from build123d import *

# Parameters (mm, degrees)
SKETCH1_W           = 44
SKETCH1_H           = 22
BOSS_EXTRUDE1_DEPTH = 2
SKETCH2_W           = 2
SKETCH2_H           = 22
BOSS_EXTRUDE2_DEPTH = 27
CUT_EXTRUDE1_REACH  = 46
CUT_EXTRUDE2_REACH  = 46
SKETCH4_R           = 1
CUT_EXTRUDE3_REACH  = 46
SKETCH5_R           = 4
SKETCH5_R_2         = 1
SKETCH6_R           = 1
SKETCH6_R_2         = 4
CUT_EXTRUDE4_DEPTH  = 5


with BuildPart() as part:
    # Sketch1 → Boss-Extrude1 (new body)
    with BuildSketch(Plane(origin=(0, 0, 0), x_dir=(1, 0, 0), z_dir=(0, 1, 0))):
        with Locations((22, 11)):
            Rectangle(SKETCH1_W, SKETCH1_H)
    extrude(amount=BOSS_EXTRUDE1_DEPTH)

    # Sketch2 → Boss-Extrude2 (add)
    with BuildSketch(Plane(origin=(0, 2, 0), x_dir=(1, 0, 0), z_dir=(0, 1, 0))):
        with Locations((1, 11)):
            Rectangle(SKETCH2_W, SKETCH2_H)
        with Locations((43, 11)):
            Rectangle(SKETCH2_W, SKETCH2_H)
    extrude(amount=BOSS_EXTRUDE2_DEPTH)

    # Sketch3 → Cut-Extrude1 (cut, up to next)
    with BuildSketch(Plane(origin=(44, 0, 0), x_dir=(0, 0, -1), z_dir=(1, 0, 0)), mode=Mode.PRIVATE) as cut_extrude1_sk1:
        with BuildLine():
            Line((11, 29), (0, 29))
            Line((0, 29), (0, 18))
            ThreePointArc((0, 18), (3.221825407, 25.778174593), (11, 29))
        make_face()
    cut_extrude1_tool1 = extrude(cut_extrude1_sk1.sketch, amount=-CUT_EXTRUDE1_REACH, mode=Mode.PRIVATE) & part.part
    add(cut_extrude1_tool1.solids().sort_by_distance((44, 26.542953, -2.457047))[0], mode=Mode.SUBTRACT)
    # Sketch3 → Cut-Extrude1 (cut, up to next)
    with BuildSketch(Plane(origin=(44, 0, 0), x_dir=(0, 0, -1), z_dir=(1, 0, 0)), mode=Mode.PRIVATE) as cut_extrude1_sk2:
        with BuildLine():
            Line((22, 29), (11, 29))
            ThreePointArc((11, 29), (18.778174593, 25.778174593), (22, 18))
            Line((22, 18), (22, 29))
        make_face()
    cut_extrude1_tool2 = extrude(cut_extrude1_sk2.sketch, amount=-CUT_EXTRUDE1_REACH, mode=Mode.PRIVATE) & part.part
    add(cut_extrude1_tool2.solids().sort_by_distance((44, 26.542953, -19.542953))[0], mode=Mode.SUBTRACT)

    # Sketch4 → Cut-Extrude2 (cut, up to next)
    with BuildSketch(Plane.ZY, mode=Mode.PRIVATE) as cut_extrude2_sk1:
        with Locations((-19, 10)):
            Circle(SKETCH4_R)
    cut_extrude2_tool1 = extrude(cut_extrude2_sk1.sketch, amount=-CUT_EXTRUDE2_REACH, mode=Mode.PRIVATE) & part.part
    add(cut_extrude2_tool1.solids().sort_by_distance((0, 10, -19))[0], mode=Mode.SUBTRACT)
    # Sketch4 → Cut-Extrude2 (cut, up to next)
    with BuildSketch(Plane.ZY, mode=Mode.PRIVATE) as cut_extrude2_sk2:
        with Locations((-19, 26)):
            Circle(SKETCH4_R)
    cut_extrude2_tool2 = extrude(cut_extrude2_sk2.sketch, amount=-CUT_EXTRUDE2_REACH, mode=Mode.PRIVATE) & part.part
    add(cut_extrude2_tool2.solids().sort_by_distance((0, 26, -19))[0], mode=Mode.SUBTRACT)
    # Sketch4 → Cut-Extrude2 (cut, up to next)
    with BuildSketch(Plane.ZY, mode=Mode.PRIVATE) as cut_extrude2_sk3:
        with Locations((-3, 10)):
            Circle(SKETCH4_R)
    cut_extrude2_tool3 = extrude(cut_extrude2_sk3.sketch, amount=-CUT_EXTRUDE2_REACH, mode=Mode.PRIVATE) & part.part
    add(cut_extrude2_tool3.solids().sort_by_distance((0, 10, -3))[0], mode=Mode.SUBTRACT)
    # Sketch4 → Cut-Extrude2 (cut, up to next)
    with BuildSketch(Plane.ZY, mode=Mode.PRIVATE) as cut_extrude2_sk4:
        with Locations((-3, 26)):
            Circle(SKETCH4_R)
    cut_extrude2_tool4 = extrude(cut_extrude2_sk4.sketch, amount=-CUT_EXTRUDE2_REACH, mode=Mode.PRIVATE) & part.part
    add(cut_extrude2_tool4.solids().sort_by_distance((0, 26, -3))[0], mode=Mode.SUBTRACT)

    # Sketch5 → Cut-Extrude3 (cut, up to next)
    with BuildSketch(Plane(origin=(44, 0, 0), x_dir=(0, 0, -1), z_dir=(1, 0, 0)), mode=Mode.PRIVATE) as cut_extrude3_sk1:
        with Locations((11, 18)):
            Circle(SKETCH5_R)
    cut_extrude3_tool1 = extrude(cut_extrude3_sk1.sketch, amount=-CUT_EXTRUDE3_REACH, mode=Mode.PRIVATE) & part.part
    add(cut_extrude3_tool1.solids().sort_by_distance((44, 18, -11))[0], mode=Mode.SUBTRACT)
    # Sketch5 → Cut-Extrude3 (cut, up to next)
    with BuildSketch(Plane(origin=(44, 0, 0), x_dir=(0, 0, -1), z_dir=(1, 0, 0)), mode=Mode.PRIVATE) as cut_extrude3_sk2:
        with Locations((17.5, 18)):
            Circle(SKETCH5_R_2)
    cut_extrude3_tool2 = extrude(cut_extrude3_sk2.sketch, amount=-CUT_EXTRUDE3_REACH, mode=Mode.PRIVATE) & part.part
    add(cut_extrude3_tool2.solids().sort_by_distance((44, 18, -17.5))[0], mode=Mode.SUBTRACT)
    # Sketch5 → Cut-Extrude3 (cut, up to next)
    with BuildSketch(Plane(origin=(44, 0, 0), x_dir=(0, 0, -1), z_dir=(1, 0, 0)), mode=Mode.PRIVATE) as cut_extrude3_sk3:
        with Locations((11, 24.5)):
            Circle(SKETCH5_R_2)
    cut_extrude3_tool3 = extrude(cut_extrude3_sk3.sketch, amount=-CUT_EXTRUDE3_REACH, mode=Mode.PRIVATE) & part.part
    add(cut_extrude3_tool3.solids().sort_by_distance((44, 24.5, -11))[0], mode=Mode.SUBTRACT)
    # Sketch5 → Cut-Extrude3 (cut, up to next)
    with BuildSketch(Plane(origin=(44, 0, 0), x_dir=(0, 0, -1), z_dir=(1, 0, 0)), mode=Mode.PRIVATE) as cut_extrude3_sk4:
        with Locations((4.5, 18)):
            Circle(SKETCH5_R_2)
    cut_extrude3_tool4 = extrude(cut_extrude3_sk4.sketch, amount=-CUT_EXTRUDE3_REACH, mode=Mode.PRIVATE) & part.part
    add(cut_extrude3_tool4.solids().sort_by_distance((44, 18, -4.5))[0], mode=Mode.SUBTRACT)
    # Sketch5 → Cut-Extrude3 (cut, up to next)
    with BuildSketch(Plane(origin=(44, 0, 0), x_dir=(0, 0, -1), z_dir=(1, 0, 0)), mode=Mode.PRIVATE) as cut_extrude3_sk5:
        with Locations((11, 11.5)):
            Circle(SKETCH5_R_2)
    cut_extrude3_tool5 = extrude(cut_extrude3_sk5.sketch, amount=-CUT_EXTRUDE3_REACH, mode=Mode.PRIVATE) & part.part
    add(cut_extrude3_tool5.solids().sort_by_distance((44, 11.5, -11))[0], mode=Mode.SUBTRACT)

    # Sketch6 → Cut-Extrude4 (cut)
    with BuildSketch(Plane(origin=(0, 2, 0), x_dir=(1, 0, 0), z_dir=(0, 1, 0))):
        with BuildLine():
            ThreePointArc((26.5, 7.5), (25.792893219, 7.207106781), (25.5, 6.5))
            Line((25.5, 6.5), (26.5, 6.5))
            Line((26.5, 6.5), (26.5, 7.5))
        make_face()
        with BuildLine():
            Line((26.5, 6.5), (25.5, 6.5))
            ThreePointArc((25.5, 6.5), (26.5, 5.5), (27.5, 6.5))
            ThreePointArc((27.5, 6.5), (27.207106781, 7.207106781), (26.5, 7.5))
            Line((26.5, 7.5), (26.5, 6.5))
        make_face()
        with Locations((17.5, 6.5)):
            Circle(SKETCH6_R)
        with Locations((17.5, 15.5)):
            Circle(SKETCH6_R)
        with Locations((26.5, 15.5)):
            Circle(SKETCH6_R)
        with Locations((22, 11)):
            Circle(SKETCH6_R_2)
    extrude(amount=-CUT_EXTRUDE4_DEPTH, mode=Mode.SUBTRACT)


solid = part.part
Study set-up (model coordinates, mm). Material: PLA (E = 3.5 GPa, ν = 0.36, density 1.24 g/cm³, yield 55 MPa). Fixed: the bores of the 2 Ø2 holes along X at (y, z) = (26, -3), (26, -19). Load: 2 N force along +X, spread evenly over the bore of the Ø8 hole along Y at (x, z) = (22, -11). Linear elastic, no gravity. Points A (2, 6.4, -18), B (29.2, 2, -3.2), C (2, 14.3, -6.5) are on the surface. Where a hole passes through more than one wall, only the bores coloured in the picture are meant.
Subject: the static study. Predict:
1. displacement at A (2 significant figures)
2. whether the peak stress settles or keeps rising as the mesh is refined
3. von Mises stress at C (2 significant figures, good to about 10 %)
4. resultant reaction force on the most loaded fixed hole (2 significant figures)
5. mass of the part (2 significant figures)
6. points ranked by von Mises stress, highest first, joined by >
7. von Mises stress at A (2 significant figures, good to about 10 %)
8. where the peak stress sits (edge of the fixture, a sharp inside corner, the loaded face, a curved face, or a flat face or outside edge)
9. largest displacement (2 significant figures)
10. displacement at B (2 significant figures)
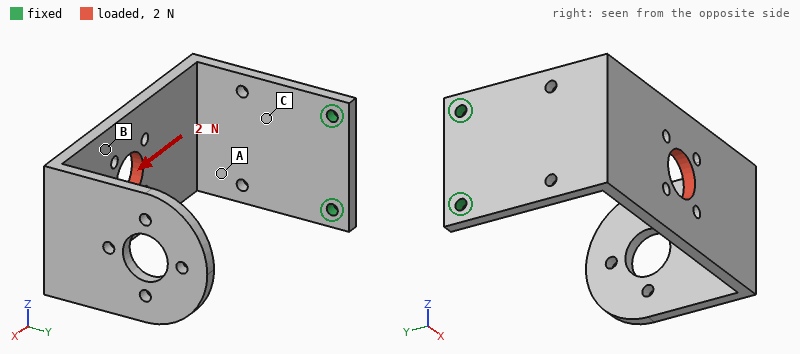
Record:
0.15 mm
keeps rising
1.7 MPa
1.0 N
4.9 g
C > A > B
0.77 MPa
edge of the fixture
0.59 mm
0.41 mm
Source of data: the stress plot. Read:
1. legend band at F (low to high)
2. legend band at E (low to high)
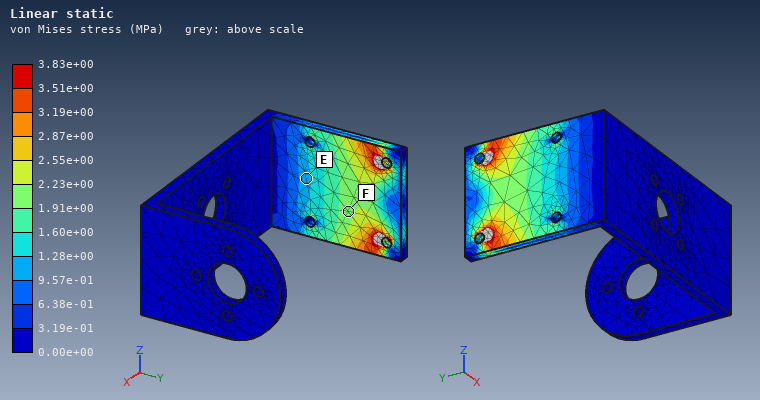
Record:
1.91e+00 to 2.23e+00 MPa
9.57e-01 to 1.28e+00 MPa
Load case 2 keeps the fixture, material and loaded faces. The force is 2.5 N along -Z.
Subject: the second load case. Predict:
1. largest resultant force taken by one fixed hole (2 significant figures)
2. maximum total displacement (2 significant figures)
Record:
5.0 N
0.59 mm
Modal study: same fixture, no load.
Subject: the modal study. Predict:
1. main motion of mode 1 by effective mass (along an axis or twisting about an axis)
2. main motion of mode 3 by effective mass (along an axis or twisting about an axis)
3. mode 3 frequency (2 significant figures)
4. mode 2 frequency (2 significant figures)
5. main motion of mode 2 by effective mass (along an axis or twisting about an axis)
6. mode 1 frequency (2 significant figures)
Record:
along Y
along X
280 Hz
160 Hz
along Z
95 Hz
